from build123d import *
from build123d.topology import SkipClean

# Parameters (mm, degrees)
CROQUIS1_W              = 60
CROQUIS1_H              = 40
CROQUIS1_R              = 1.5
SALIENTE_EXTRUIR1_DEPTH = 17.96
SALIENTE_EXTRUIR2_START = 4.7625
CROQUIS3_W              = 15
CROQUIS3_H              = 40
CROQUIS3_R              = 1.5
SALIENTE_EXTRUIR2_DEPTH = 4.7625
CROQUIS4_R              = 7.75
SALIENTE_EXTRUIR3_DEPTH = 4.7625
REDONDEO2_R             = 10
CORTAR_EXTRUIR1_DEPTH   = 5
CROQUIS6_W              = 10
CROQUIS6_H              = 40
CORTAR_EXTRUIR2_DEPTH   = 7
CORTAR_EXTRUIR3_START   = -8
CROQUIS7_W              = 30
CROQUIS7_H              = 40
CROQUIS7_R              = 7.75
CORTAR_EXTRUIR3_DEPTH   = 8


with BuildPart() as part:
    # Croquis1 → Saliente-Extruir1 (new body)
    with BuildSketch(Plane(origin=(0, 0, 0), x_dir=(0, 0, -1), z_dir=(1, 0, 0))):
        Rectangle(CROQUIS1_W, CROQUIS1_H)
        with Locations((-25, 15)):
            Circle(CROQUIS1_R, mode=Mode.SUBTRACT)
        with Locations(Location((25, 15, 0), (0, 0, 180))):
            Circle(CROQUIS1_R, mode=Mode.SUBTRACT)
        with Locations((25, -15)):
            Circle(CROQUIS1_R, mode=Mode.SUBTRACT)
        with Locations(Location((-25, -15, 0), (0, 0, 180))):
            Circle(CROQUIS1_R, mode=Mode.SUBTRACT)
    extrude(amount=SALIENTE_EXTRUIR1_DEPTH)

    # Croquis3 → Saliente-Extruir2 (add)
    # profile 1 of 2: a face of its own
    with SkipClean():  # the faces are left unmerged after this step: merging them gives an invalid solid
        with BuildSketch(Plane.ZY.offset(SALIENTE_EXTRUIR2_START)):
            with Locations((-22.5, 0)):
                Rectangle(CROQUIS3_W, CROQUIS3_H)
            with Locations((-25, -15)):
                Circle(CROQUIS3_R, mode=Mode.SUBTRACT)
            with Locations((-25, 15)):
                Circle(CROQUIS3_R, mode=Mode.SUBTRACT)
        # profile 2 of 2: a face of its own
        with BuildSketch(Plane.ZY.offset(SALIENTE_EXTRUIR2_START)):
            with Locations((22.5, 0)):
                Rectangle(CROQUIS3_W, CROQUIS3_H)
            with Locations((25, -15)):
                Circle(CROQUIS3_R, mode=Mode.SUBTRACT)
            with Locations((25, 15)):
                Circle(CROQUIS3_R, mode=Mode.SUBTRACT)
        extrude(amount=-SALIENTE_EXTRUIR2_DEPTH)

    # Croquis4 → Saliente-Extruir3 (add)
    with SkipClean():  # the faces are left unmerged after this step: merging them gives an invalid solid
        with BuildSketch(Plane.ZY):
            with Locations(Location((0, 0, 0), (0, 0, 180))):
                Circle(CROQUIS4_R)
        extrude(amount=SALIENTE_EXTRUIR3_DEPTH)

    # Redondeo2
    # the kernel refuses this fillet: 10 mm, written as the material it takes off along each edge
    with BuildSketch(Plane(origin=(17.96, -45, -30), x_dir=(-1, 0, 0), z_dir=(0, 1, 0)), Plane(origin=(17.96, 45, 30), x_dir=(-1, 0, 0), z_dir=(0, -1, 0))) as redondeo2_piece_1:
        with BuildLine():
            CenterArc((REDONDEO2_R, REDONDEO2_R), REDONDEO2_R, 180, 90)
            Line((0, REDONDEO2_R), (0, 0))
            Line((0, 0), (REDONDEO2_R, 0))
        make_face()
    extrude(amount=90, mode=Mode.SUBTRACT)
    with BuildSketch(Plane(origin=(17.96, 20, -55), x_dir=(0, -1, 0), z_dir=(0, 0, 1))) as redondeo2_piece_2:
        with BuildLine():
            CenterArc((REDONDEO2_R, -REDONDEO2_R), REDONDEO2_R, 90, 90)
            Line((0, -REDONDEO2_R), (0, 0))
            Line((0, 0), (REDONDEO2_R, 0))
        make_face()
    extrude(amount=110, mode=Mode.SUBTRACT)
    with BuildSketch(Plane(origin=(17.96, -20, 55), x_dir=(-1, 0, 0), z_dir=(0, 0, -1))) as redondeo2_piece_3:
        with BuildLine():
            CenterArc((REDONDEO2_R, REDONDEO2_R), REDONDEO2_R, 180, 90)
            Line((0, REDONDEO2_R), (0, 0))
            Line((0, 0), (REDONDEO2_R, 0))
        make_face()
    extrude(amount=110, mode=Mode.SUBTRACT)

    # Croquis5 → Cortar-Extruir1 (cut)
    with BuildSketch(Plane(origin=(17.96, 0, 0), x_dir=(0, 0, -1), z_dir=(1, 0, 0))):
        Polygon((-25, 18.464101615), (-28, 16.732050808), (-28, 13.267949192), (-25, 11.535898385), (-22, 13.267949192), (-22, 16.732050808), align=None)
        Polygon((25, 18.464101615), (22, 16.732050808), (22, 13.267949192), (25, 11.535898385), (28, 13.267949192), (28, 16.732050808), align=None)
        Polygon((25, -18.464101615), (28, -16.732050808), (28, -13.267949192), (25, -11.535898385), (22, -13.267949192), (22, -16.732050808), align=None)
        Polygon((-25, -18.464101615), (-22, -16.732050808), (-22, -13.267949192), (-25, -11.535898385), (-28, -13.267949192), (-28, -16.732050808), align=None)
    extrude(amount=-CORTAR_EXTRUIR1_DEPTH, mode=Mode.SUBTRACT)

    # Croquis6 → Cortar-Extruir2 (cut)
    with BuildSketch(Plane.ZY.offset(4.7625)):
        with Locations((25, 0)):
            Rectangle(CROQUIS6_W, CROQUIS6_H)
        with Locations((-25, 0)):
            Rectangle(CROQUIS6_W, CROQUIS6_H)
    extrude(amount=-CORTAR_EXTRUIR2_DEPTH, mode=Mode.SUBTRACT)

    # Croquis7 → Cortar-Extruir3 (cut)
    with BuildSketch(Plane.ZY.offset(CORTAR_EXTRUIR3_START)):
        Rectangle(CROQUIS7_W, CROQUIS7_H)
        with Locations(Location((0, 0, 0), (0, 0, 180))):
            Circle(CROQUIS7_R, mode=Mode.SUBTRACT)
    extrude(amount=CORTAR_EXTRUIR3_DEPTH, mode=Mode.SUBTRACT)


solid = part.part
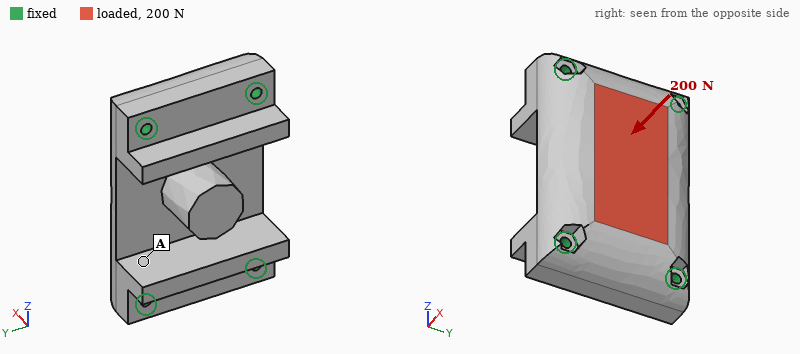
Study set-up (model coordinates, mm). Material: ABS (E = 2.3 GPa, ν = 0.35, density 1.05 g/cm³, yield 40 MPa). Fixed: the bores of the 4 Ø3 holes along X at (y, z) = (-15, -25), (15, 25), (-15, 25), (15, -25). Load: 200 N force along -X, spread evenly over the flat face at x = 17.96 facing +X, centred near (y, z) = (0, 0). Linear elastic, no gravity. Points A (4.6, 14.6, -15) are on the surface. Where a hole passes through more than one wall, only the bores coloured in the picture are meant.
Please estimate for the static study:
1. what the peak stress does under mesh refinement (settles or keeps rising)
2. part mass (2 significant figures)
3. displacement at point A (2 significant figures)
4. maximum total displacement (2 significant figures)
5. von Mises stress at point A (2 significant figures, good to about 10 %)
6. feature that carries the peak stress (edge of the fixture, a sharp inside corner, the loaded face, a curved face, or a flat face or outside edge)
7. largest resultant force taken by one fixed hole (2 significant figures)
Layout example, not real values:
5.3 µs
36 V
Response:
keeps rising
33 g
7.0 µm
17 µm
0.40 MPa
edge of the fixture
65 N
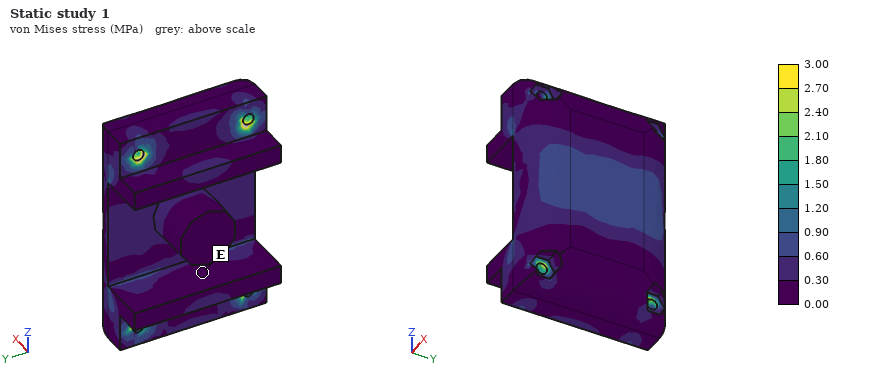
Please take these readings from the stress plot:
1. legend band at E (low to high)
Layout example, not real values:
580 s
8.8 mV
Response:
0.00 to 0.30 MPa
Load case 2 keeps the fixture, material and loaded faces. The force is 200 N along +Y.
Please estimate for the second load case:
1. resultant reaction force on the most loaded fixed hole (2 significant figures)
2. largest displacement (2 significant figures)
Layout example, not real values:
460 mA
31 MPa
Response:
70 N
9.5 µm
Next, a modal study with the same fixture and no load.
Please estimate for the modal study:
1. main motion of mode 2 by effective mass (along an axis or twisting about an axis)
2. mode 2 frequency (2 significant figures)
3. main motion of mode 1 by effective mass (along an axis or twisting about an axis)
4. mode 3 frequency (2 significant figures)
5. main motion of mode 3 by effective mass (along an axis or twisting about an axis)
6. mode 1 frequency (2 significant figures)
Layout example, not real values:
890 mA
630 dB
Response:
along Y
5200 Hz
along X
6000 Hz
along Z
4100 Hz
